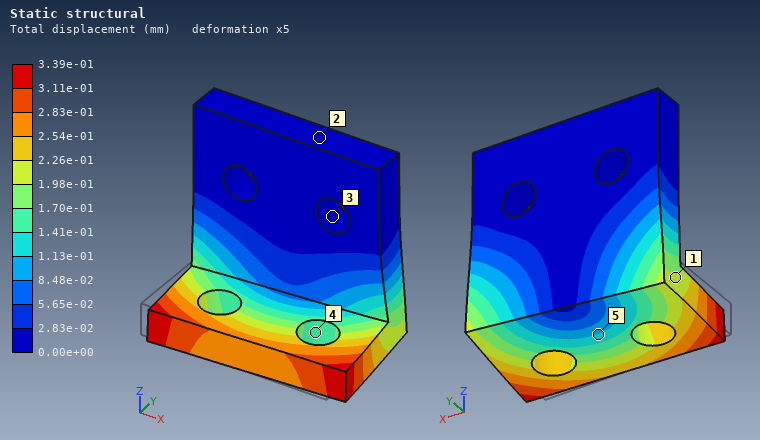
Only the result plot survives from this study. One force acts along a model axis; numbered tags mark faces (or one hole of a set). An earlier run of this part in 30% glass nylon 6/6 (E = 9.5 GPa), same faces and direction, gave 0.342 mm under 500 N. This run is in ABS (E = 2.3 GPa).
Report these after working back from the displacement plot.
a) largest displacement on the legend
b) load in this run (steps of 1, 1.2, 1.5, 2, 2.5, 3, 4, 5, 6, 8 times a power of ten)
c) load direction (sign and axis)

3.39e-01 mm
120 N
+X
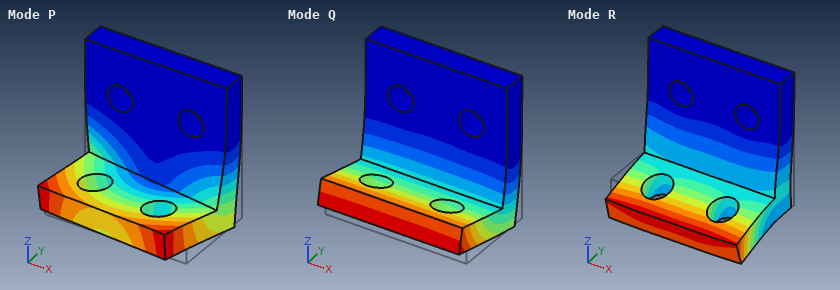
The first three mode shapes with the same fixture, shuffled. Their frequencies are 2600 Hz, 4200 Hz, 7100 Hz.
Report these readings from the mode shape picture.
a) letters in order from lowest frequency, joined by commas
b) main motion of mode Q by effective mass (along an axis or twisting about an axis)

Q, P, R
along Y
